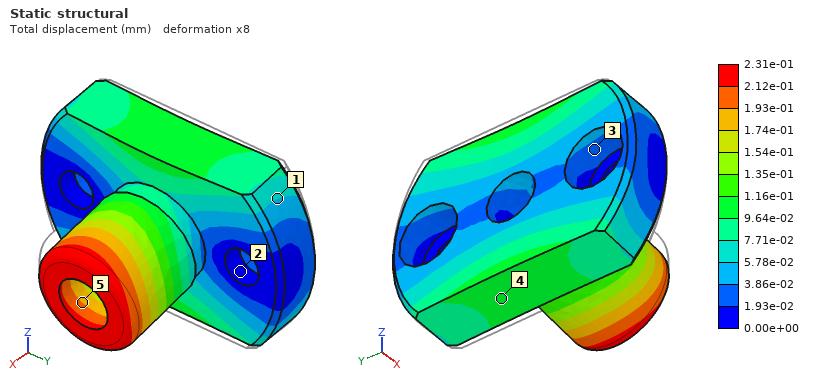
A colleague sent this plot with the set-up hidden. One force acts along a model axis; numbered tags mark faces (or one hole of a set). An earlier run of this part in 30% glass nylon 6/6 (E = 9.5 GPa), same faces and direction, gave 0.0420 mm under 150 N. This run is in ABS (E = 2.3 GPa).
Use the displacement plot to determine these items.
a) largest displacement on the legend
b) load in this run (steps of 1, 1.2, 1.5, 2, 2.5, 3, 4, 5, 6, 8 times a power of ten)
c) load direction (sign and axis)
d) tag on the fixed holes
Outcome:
2.31e-01 mm
200 N
-Z
2
